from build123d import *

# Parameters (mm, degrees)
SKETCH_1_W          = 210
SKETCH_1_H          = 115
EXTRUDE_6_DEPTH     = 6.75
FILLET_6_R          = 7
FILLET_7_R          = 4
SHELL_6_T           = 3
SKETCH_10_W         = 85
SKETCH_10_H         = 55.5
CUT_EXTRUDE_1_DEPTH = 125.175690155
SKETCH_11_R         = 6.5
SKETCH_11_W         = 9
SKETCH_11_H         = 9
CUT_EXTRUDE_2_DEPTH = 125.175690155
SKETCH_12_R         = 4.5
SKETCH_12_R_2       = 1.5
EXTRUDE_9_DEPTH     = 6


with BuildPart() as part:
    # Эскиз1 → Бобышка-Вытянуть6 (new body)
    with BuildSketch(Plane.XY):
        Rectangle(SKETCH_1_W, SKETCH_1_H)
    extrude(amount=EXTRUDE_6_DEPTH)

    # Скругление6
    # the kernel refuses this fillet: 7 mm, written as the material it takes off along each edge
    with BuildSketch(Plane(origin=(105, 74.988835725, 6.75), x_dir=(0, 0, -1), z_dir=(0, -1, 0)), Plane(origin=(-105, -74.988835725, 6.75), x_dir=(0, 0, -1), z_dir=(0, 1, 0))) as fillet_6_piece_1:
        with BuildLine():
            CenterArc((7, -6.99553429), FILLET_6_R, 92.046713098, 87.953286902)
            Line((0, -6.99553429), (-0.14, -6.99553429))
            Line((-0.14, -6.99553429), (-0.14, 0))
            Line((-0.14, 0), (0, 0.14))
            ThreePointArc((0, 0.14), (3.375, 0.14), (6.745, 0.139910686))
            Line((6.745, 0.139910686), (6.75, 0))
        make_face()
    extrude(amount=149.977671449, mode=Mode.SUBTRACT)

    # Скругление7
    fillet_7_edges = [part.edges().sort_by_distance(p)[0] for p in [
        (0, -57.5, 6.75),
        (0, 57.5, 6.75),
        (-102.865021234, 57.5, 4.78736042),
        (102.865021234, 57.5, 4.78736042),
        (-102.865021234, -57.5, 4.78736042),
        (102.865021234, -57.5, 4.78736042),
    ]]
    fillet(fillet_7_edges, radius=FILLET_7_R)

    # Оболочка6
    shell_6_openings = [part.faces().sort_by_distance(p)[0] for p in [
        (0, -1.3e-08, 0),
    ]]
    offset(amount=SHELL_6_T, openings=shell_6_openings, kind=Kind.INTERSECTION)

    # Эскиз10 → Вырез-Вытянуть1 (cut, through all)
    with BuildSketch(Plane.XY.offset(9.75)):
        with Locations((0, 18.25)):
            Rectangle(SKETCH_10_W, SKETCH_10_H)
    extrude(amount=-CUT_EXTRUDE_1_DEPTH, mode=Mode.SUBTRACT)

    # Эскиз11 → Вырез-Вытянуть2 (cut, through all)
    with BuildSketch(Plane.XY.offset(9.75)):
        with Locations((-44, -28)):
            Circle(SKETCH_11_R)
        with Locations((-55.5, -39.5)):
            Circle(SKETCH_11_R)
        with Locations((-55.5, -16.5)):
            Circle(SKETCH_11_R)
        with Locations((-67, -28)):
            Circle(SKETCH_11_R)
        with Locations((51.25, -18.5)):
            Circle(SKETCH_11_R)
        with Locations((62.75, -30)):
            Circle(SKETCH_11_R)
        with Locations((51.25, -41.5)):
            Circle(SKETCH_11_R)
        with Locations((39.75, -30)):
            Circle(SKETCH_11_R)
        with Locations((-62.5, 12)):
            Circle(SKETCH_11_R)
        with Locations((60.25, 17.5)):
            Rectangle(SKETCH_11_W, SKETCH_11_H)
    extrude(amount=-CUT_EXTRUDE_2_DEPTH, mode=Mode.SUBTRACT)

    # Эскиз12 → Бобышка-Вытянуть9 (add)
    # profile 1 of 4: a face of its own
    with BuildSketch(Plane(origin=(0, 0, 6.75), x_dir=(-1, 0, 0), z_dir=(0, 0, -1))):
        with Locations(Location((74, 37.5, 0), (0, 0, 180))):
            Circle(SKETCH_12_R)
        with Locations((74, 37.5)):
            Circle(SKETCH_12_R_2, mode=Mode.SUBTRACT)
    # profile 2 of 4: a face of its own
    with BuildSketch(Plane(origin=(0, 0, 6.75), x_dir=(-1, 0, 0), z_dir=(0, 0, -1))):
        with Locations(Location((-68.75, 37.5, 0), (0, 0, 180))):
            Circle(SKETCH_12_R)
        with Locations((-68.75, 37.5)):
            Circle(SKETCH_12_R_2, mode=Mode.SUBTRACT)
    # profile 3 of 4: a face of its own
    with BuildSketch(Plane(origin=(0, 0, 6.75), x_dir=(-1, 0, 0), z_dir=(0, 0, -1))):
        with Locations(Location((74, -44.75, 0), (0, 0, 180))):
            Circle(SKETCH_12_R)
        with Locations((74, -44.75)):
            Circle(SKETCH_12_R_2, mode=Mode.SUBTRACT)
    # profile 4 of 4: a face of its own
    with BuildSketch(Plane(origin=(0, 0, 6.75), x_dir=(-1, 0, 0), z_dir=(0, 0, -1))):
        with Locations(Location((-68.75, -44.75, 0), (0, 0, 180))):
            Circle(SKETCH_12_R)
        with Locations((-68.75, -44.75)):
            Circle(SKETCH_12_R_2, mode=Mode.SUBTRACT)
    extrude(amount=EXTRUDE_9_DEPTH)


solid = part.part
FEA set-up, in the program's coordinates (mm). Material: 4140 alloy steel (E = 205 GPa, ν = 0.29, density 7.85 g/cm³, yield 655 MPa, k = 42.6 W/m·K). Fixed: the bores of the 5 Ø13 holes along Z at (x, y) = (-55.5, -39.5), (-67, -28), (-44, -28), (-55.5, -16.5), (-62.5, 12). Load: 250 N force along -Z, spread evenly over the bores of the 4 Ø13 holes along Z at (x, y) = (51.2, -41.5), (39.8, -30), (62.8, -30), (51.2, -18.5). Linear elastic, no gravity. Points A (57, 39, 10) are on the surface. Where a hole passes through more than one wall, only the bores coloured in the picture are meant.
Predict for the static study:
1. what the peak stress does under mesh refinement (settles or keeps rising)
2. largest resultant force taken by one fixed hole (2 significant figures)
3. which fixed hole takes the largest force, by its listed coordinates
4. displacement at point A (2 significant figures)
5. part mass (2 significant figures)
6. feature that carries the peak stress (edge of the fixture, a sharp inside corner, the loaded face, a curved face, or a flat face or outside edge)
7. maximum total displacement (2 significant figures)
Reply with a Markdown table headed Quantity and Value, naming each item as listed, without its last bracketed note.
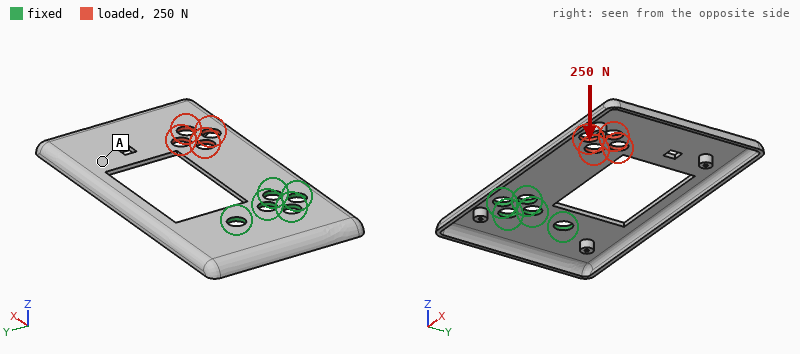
| Quantity | Value |
|---|---|
| what the peak stress does under mesh refinement | keeps rising |
| largest resultant force taken by one fixed hole | 820 N |
| which fixed hole takes the largest force, by its listed coordinates | (-44, -28) |
| displacement at point A | 0.72 mm |
| part mass | 540 g |
| feature that carries the peak stress | edge of the fixture |
| maximum total displacement | 1.3 mm |
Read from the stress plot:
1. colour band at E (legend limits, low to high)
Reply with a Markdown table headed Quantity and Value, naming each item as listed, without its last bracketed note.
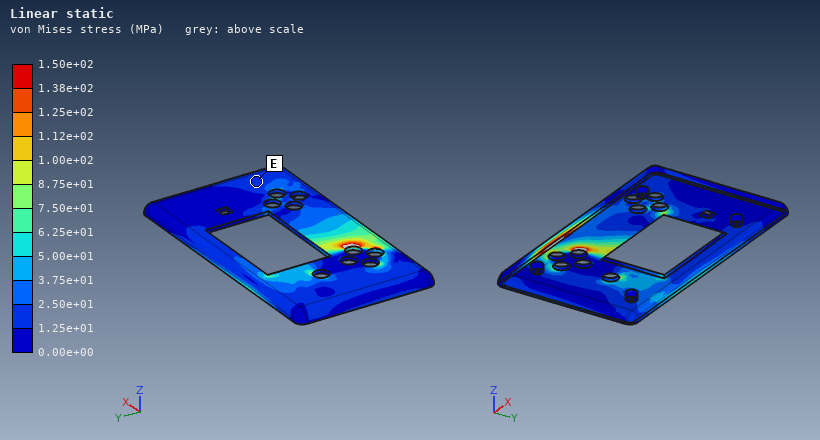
| Quantity | Value |
|---|---|
| colour band at E | 1.25e+01 to 2.50e+01 MPa |
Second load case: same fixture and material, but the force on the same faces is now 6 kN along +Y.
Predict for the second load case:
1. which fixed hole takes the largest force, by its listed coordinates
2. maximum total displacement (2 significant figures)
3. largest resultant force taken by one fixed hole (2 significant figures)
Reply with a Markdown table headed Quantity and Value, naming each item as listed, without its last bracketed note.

| Quantity | Value |
|---|---|
| which fixed hole takes the largest force, by its listed coordinates | (-55.5, -39.5) |
| maximum total displacement | 0.59 mm |
| largest resultant force taken by one fixed hole | 10 kN |
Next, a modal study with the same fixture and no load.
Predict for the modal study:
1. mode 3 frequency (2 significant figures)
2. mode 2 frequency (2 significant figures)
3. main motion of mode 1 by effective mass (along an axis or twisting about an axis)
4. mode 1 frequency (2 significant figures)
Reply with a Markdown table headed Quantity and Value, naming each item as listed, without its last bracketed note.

| Quantity | Value |
|---|---|
| mode 3 frequency | 840 Hz |
| mode 2 frequency | 280 Hz |
| main motion of mode 1 by effective mass | along Z |
| mode 1 frequency | 130 Hz |
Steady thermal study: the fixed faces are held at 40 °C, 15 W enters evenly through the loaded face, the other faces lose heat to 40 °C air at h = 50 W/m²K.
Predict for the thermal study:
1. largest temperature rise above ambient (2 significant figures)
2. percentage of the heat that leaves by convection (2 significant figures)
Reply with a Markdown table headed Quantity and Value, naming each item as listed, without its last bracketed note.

| Quantity | Value |
|---|---|
| largest temperature rise above ambient | 47 K |
| percentage of the heat that leaves by convection | 94 % |
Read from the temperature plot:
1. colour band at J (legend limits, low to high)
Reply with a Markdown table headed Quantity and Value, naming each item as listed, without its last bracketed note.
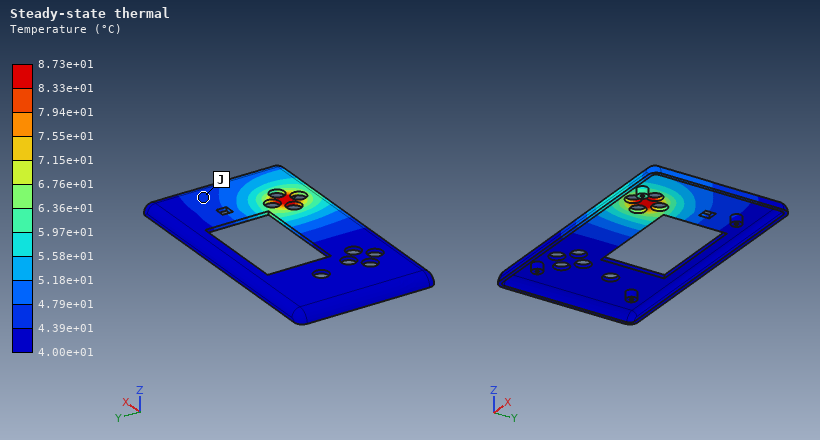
| Quantity | Value |
|---|---|
| colour band at J | 4.39e+01 to 4.79e+01 °C |
